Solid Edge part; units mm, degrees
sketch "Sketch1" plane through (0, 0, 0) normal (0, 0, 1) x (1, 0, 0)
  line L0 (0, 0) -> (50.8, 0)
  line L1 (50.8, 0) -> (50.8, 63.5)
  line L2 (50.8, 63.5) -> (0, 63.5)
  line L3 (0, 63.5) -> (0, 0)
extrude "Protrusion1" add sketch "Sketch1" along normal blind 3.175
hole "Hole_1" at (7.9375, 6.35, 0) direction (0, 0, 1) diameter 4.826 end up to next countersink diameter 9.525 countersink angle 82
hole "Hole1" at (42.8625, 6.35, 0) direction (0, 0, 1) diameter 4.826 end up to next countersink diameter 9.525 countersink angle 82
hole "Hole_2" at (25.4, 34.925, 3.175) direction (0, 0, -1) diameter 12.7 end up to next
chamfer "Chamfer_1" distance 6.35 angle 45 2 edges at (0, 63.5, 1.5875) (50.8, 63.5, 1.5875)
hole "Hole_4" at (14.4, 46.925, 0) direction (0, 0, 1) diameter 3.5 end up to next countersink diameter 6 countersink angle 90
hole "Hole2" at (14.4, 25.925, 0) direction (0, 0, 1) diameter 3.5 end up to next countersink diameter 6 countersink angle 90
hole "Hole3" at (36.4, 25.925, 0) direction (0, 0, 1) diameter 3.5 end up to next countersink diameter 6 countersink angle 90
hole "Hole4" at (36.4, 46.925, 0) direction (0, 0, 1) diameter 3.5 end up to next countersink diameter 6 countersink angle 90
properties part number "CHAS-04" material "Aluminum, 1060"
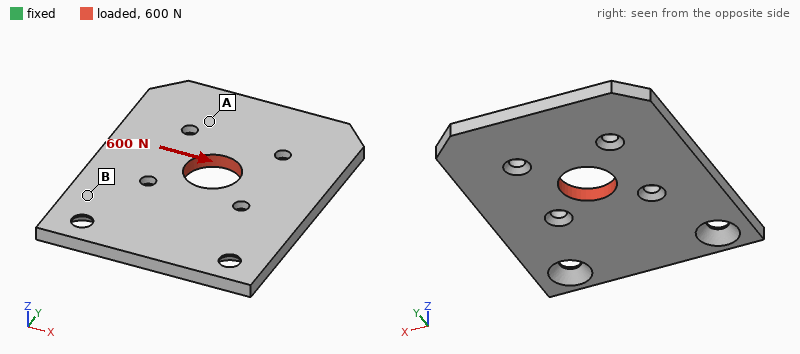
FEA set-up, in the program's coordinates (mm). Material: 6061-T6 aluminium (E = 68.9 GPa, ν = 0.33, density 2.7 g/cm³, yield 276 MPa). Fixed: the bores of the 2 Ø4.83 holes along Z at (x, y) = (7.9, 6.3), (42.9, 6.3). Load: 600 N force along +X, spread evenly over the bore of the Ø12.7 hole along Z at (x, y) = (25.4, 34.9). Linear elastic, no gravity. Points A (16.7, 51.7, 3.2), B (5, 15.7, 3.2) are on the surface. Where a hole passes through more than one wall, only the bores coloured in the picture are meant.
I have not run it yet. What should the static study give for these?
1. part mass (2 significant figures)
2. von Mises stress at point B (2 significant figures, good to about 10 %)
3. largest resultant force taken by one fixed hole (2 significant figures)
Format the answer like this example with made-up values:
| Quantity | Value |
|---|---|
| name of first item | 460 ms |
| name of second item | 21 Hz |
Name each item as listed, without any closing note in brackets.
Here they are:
| Quantity | Value |
|---|---|
| part mass | 25 g |
| von Mises stress at point B | 15 MPa |
| largest resultant force taken by one fixed hole | 550 N |
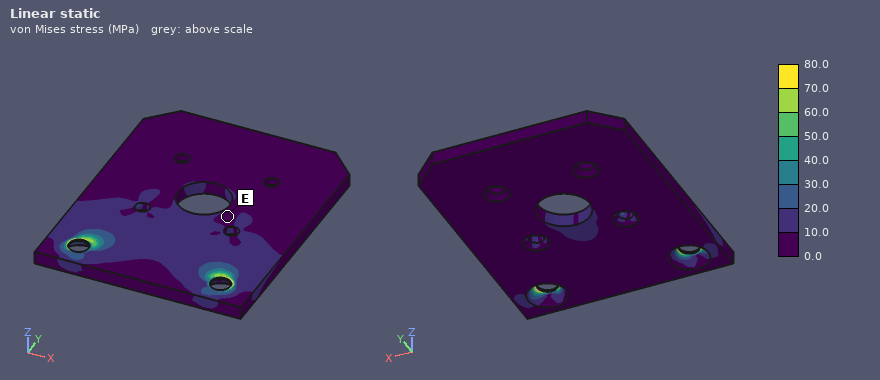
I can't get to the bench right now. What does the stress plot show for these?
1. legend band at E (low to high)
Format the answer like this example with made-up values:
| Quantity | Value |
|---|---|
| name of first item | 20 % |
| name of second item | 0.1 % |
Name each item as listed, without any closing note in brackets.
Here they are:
| Quantity | Value |
|---|---|
| legend band at E | 0.0 to 10.0 MPa |
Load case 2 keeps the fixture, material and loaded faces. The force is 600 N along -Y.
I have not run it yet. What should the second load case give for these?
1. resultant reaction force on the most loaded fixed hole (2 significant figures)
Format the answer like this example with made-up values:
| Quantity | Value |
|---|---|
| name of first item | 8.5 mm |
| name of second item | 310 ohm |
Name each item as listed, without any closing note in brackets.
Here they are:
| Quantity | Value |
|---|---|
| resultant reaction force on the most loaded fixed hole | 300 N |
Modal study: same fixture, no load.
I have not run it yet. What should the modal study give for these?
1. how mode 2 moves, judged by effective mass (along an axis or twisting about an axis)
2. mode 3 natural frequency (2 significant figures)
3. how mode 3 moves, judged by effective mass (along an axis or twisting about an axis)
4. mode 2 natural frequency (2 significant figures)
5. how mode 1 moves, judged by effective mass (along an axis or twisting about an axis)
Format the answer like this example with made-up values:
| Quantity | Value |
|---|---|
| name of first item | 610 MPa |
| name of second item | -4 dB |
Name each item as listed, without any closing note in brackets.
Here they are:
| Quantity | Value |
|---|---|
| how mode 2 moves, judged by effective mass | twisting about Y |
| mode 3 natural frequency | 3800 Hz |
| how mode 3 moves, judged by effective mass | along Z |
| mode 2 natural frequency | 1900 Hz |
| how mode 1 moves, judged by effective mass | along Z |
